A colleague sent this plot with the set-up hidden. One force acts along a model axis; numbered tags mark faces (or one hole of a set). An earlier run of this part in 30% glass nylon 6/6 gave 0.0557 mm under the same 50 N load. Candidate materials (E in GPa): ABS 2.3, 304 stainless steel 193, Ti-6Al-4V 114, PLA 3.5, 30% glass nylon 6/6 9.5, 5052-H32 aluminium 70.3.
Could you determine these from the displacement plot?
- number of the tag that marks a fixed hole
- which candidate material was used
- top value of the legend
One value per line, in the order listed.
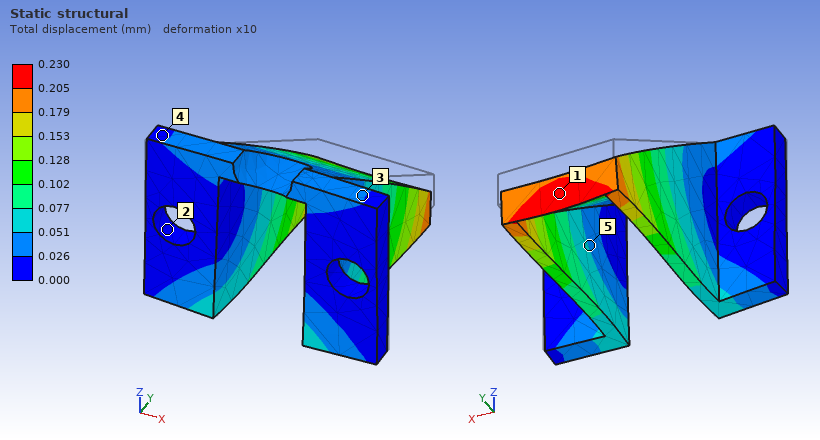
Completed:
2
ABS
0.230 mm
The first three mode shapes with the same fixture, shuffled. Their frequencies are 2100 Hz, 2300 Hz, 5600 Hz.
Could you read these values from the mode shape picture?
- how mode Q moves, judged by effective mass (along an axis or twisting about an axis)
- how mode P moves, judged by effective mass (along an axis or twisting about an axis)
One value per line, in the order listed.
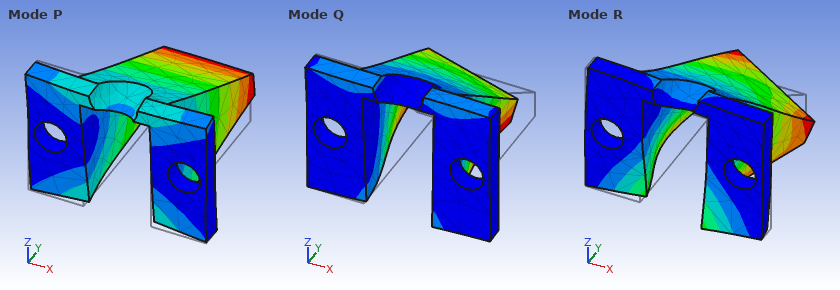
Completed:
along X
along Z
